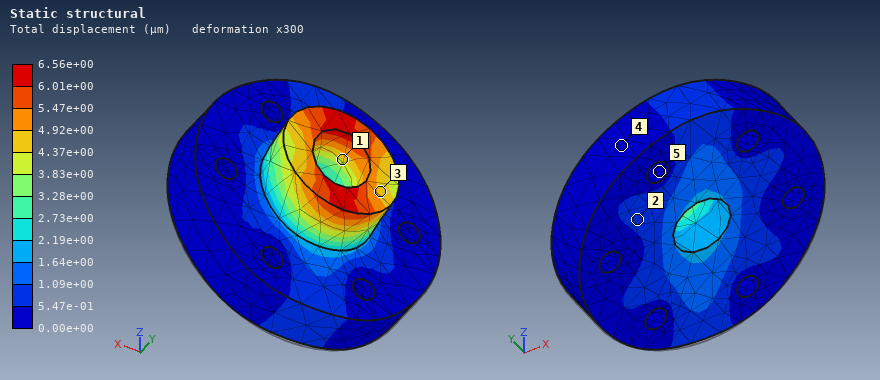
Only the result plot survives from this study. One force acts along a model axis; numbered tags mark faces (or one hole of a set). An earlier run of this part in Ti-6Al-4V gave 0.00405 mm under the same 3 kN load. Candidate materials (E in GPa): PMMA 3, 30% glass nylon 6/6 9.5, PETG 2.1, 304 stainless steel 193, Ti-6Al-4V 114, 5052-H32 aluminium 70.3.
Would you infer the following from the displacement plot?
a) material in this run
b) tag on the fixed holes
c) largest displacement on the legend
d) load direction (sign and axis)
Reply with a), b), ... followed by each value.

a) 5052-H32 aluminium
b) 5
c) 6.56e+00 µm
d) +Z
